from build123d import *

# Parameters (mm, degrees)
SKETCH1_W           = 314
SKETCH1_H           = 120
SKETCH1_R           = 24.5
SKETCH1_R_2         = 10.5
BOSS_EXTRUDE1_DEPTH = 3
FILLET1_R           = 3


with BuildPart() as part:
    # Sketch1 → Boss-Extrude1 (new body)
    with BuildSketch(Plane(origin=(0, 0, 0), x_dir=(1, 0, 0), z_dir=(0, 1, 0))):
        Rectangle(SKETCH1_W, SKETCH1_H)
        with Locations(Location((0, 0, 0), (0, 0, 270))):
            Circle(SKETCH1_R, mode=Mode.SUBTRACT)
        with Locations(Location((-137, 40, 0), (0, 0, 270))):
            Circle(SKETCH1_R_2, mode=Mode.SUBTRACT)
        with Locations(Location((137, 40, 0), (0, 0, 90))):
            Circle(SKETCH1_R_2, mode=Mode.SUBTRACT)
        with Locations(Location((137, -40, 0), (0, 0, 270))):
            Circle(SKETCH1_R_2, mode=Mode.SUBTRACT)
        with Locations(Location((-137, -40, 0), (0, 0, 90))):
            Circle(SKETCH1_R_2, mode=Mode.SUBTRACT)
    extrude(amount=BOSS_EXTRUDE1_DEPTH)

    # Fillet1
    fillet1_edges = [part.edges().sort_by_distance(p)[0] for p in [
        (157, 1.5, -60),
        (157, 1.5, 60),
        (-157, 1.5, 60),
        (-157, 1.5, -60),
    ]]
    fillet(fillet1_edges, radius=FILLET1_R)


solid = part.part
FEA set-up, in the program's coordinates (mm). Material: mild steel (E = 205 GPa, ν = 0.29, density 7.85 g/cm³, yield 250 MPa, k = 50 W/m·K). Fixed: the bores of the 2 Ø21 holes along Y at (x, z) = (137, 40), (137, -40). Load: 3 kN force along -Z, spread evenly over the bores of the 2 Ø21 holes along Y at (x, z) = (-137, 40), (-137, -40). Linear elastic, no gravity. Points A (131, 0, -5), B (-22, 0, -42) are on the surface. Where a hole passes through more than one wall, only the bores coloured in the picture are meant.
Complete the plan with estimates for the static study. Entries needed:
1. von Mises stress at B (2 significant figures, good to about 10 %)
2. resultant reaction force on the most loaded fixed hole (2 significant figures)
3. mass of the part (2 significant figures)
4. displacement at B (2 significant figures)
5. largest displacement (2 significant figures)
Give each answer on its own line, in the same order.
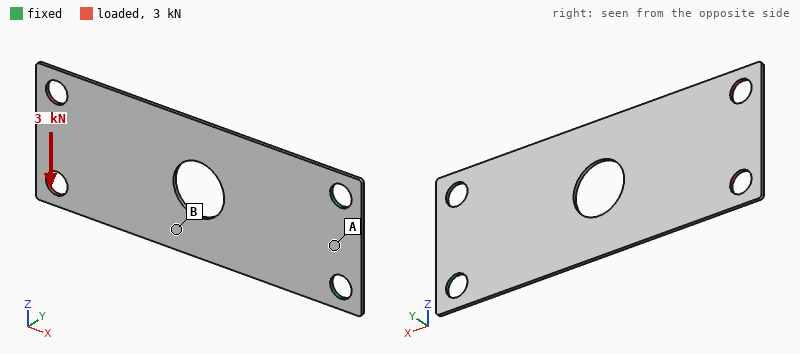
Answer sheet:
34 MPa
9.4 kN
810 g
0.13 mm
0.31 mm
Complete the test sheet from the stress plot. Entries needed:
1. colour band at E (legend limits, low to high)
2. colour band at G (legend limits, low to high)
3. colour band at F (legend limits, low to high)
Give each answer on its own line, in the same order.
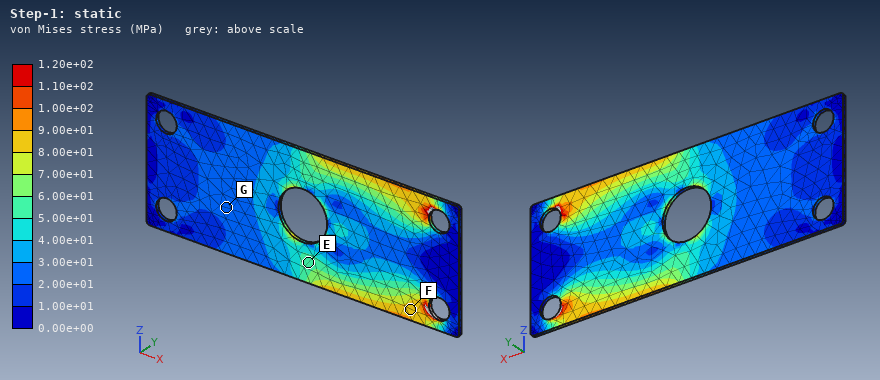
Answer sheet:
5.00e+01 to 6.00e+01 MPa
2.00e+01 to 3.00e+01 MPa
8.00e+01 to 9.00e+01 MPa
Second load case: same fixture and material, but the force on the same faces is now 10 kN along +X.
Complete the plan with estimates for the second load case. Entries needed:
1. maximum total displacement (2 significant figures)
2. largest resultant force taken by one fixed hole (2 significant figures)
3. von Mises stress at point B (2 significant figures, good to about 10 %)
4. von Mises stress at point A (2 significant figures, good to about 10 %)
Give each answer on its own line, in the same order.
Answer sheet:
55 µm
5.0 kN
43 MPa
8.3 MPa
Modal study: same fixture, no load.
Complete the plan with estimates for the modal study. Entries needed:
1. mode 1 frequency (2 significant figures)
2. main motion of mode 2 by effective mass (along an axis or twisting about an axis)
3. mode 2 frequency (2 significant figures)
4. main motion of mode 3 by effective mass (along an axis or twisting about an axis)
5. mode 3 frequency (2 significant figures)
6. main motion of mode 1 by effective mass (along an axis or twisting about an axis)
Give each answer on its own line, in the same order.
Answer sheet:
31 Hz
twisting about X
150 Hz
along Y
190 Hz
along Y
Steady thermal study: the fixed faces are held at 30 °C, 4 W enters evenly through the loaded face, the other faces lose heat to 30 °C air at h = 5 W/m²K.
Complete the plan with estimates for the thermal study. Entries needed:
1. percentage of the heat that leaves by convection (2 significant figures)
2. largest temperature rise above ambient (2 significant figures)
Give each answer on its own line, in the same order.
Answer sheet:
83 %
28 K
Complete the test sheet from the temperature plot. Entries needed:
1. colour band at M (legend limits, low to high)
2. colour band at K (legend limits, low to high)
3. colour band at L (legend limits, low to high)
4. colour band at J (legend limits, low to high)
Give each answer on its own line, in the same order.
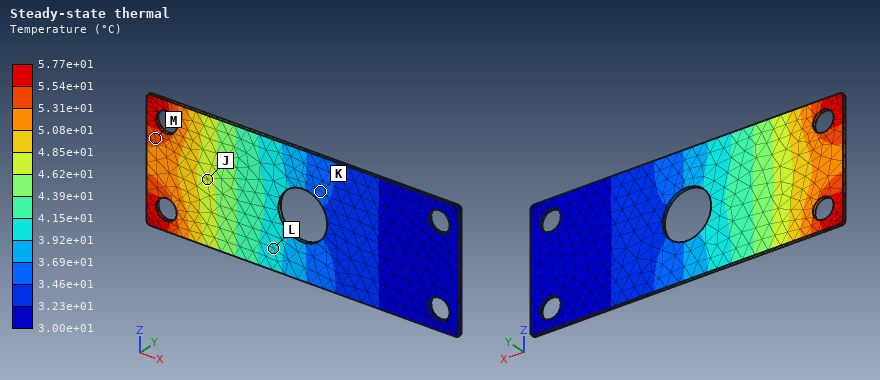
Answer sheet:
5.31e+01 to 5.54e+01 °C
3.46e+01 to 3.69e+01 °C
3.92e+01 to 4.15e+01 °C
4.62e+01 to 4.85e+01 °C
